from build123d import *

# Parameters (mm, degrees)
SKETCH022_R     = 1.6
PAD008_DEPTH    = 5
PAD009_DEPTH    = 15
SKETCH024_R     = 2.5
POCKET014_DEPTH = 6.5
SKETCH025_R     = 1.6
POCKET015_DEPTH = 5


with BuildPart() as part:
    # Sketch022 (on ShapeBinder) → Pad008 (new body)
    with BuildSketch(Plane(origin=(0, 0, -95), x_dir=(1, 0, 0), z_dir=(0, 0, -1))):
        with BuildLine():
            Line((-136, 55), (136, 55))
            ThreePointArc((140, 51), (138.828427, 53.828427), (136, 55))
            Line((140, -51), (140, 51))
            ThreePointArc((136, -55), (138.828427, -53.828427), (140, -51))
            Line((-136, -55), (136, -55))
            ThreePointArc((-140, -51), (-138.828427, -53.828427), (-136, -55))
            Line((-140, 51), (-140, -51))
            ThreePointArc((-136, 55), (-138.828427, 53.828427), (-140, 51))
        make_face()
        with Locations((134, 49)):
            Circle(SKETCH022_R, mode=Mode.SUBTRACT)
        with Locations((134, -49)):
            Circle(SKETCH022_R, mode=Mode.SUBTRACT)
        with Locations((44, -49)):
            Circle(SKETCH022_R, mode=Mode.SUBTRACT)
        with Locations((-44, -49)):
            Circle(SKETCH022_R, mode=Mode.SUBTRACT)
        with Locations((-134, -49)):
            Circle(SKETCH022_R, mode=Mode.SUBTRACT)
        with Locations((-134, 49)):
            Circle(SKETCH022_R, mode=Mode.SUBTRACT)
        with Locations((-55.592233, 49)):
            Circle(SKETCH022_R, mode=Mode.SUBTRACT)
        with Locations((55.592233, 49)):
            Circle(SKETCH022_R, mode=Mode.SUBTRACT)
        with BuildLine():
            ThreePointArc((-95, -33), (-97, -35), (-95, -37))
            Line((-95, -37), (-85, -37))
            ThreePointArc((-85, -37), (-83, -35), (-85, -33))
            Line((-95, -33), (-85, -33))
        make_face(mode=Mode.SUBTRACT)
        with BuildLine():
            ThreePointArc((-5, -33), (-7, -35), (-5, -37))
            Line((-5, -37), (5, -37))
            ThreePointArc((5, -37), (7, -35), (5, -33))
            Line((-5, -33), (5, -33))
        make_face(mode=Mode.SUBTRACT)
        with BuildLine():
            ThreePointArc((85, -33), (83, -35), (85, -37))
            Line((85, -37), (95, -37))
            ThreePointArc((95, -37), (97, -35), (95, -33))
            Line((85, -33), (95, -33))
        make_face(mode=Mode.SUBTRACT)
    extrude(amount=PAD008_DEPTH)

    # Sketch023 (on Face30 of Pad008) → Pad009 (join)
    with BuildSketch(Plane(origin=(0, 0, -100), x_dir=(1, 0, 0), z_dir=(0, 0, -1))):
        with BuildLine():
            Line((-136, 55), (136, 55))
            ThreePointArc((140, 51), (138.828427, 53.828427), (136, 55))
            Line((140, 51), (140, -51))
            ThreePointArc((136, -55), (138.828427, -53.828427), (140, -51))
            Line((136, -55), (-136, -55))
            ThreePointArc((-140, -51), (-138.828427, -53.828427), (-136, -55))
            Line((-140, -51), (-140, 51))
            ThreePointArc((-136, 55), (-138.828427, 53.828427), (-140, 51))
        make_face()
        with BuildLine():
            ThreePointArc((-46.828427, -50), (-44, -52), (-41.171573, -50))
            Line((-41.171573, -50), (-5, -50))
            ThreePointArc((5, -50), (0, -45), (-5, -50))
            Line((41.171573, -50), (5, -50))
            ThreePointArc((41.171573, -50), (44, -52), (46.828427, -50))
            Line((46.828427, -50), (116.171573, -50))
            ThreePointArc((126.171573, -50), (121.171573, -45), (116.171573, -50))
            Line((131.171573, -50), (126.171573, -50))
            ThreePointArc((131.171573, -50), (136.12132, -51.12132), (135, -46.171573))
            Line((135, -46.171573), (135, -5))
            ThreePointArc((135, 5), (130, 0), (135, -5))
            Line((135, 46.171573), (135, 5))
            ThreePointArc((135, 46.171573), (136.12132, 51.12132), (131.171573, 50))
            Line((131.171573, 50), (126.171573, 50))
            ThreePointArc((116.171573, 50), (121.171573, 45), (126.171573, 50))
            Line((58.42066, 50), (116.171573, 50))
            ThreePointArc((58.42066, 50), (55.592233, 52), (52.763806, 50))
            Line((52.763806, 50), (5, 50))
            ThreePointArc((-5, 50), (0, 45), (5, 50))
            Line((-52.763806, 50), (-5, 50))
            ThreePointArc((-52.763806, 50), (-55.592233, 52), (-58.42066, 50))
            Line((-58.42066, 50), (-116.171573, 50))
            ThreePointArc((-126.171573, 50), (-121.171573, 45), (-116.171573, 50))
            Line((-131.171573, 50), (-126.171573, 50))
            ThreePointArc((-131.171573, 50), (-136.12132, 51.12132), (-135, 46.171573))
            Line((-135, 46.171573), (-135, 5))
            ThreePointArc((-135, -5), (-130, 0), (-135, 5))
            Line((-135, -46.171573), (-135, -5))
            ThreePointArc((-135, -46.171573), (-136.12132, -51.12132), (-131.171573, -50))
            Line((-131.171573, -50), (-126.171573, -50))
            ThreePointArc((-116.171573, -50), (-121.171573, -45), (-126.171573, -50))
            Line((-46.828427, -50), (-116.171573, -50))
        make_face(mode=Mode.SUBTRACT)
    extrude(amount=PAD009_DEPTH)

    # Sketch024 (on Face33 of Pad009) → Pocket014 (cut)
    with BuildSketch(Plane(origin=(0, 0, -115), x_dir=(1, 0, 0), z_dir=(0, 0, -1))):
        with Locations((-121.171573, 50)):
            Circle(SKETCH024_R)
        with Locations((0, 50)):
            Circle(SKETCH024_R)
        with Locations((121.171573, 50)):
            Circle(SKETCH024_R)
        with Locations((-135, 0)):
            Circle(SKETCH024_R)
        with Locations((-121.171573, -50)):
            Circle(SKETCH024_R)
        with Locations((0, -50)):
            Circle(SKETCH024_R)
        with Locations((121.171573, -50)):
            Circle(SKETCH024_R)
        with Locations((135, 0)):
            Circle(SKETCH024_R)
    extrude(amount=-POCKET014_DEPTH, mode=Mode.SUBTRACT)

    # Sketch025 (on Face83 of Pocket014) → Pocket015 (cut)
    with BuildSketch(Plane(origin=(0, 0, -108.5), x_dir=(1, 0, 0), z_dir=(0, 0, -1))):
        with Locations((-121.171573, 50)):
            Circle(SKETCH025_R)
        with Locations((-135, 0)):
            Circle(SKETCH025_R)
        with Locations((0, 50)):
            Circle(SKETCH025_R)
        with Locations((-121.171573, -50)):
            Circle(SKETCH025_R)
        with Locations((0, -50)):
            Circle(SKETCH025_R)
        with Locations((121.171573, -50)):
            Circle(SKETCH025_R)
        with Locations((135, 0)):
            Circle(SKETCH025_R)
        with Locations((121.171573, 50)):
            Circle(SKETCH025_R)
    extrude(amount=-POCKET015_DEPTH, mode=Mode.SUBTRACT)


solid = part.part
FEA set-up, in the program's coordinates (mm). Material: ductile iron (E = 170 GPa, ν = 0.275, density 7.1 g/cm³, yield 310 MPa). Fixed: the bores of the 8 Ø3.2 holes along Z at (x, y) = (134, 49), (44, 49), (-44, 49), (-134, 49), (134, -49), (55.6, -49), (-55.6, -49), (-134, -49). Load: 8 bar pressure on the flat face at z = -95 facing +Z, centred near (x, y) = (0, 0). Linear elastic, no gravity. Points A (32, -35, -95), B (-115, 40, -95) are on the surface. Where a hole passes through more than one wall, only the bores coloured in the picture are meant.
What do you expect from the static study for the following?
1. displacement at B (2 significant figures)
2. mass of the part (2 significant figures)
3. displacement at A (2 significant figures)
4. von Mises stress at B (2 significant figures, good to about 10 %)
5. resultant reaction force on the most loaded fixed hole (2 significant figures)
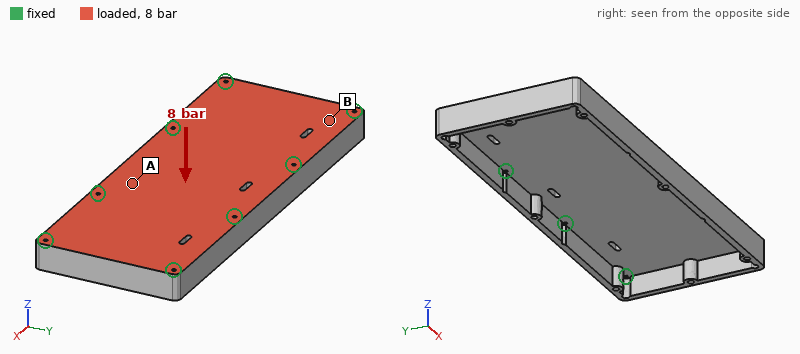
0.041 mm
1.5 kg
0.11 mm
46 MPa
4.5 kN
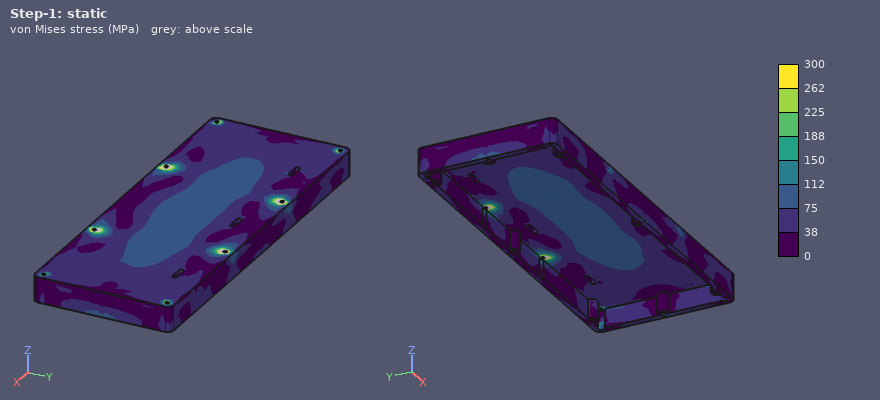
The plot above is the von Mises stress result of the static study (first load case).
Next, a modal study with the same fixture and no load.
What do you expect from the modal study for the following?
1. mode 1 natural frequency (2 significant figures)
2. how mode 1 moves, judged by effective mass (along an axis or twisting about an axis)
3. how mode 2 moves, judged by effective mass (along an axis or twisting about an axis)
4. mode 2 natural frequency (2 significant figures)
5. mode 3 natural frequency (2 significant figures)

1800 Hz
along Z
twisting about Y
2300 Hz
2500 Hz
